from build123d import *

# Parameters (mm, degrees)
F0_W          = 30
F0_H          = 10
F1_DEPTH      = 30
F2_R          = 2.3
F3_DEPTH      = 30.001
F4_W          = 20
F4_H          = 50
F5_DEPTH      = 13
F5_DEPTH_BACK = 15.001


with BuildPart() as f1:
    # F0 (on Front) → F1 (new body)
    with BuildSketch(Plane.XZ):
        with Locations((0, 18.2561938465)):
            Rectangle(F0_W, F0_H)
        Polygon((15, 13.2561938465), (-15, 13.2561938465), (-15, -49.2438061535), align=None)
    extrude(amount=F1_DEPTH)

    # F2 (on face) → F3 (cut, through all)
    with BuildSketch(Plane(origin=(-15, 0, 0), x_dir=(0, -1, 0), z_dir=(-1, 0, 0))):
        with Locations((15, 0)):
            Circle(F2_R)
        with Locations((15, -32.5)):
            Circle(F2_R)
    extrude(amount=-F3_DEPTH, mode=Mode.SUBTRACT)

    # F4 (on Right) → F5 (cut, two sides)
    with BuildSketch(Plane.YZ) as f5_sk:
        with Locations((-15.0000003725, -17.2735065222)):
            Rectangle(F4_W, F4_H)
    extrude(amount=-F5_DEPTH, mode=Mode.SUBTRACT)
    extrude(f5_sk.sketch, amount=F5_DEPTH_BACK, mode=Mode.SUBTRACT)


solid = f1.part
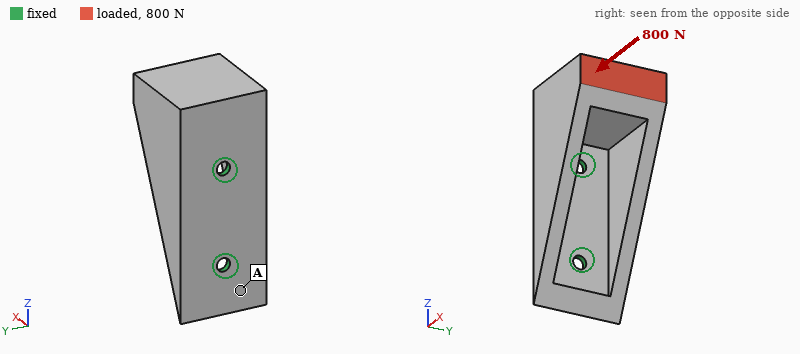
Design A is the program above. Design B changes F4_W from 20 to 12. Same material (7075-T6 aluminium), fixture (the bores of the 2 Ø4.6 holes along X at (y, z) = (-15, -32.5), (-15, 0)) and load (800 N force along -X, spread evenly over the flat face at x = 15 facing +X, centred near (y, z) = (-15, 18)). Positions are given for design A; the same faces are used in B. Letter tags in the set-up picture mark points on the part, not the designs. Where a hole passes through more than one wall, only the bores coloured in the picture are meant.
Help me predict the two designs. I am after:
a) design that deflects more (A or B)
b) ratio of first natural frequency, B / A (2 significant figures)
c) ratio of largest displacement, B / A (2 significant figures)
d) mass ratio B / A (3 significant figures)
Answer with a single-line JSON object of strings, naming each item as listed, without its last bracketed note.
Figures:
{"design that deflects more": "A", "ratio of first natural frequency, B / A": "1.1", "ratio of largest displacement, B / A": "0.51", "mass ratio B / A": "1.23"}
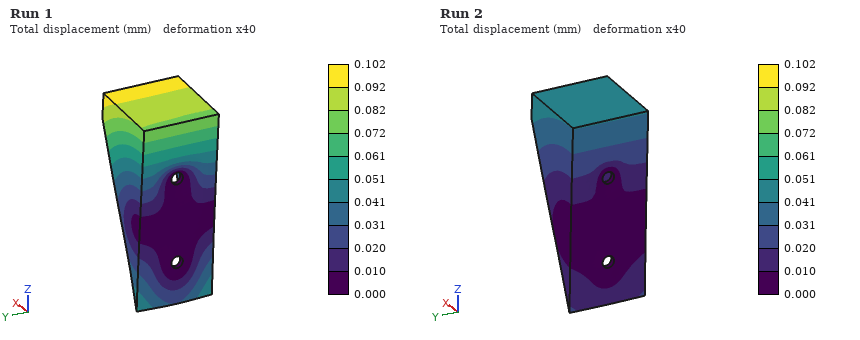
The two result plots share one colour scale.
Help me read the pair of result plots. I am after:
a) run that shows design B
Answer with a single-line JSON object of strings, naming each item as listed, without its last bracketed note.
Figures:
{"run that shows design B": "Run 2"}
